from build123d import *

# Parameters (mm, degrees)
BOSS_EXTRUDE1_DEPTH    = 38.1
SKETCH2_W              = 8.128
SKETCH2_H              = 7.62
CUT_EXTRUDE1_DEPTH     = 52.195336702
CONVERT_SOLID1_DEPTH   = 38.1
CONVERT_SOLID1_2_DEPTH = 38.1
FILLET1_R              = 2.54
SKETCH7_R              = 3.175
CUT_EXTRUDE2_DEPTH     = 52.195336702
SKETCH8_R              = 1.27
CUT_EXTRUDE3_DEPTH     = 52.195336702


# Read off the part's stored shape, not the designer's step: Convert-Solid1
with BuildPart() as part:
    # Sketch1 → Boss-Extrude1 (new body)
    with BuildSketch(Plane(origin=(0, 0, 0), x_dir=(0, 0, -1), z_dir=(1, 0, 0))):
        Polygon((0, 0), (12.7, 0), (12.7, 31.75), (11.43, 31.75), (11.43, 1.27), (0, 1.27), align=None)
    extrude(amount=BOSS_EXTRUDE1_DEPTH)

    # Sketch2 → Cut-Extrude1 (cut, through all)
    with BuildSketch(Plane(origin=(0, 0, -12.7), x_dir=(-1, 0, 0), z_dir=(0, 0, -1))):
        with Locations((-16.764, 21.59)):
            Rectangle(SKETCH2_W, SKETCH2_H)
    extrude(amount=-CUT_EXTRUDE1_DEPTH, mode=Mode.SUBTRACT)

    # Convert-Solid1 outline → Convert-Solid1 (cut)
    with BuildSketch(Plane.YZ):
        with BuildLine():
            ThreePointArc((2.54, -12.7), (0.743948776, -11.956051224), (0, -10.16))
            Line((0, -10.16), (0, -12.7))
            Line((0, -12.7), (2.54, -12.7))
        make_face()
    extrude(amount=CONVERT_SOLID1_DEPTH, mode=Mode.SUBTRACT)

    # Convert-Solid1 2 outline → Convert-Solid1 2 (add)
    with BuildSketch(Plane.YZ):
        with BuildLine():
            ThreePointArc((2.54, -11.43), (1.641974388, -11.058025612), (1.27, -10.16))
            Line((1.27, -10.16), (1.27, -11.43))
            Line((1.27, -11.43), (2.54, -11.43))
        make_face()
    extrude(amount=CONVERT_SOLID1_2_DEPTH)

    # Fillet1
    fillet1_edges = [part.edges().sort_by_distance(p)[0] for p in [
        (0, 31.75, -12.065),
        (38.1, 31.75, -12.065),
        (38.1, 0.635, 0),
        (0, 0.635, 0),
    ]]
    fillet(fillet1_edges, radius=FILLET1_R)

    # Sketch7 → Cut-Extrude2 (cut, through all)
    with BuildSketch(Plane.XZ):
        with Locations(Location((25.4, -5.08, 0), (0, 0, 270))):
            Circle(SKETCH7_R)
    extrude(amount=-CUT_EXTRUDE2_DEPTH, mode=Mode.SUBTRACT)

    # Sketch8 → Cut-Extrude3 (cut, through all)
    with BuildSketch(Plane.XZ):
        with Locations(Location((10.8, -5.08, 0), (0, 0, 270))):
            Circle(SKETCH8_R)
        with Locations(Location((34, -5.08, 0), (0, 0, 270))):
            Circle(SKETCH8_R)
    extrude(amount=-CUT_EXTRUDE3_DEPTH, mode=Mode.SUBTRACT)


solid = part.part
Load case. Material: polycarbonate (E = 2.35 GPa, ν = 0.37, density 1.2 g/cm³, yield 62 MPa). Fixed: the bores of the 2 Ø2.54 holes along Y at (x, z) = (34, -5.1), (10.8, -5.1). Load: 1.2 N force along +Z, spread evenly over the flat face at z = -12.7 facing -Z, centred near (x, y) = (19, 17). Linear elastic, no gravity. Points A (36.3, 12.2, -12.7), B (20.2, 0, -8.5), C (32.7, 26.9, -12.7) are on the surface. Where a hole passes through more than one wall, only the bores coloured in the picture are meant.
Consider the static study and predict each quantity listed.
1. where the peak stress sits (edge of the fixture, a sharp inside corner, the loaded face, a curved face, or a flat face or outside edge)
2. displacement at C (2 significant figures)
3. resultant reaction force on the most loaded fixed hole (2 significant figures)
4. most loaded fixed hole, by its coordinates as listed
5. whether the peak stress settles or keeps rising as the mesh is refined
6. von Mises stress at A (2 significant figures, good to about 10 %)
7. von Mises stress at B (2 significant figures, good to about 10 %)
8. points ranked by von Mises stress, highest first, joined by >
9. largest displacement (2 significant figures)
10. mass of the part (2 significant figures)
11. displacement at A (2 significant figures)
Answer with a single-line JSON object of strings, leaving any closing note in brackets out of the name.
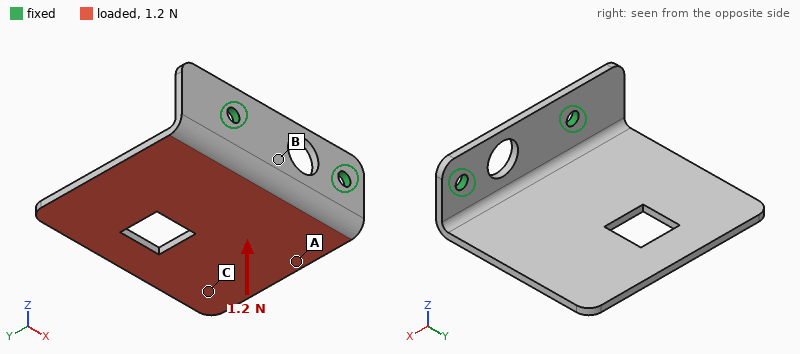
{"where the peak stress sits": "edge of the fixture", "displacement at C": "0.46 mm", "resultant reaction force on the most loaded fixed hole": "0.78 N", "most loaded fixed hole, by its coordinates as listed": "(10.8, -5.1)", "whether the peak stress settles or keeps rising as the mesh is refined": "keeps rising", "von Mises stress at A": "0.81 MPa", "von Mises stress at B": "1.5 MPa", "points ranked by von Mises stress, highest first, joined by >": "B > A > C", "largest displacement": "0.56 mm", "mass of the part": "2.3 g", "displacement at A": "0.16 mm"}
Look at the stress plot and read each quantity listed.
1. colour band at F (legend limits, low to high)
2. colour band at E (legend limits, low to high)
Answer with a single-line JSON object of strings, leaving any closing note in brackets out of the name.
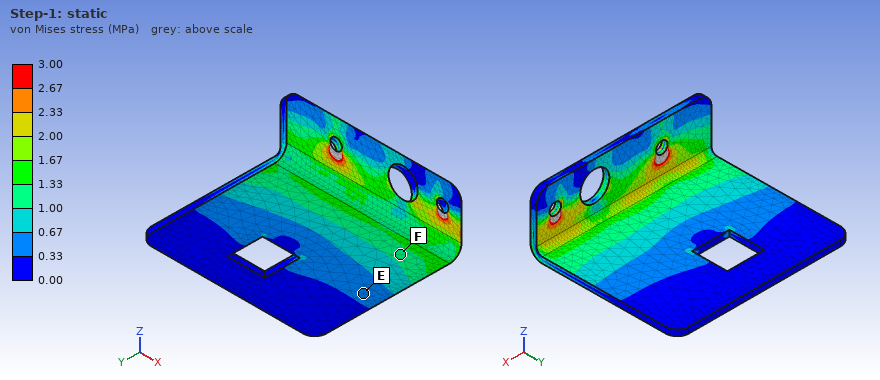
{"colour band at F": "1.00 to 1.33 MPa", "colour band at E": "0.33 to 0.67 MPa"}
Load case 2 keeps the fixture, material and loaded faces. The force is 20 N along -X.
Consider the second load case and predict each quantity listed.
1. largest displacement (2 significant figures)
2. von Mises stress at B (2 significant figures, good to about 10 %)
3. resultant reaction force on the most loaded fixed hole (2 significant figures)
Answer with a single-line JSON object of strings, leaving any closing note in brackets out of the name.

{"largest displacement": "0.60 mm", "von Mises stress at B": "2.5 MPa", "resultant reaction force on the most loaded fixed hole": "18 N"}
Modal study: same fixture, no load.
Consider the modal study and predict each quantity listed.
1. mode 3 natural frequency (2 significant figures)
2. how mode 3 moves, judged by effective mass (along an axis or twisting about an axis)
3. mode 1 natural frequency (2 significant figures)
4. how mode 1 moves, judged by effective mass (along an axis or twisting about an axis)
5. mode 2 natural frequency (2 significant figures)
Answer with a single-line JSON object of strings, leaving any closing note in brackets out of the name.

{"mode 3 natural frequency": "960 Hz", "how mode 3 moves, judged by effective mass": "along X", "mode 1 natural frequency": "230 Hz", "how mode 1 moves, judged by effective mass": "along Z", "mode 2 natural frequency": "520 Hz"}
